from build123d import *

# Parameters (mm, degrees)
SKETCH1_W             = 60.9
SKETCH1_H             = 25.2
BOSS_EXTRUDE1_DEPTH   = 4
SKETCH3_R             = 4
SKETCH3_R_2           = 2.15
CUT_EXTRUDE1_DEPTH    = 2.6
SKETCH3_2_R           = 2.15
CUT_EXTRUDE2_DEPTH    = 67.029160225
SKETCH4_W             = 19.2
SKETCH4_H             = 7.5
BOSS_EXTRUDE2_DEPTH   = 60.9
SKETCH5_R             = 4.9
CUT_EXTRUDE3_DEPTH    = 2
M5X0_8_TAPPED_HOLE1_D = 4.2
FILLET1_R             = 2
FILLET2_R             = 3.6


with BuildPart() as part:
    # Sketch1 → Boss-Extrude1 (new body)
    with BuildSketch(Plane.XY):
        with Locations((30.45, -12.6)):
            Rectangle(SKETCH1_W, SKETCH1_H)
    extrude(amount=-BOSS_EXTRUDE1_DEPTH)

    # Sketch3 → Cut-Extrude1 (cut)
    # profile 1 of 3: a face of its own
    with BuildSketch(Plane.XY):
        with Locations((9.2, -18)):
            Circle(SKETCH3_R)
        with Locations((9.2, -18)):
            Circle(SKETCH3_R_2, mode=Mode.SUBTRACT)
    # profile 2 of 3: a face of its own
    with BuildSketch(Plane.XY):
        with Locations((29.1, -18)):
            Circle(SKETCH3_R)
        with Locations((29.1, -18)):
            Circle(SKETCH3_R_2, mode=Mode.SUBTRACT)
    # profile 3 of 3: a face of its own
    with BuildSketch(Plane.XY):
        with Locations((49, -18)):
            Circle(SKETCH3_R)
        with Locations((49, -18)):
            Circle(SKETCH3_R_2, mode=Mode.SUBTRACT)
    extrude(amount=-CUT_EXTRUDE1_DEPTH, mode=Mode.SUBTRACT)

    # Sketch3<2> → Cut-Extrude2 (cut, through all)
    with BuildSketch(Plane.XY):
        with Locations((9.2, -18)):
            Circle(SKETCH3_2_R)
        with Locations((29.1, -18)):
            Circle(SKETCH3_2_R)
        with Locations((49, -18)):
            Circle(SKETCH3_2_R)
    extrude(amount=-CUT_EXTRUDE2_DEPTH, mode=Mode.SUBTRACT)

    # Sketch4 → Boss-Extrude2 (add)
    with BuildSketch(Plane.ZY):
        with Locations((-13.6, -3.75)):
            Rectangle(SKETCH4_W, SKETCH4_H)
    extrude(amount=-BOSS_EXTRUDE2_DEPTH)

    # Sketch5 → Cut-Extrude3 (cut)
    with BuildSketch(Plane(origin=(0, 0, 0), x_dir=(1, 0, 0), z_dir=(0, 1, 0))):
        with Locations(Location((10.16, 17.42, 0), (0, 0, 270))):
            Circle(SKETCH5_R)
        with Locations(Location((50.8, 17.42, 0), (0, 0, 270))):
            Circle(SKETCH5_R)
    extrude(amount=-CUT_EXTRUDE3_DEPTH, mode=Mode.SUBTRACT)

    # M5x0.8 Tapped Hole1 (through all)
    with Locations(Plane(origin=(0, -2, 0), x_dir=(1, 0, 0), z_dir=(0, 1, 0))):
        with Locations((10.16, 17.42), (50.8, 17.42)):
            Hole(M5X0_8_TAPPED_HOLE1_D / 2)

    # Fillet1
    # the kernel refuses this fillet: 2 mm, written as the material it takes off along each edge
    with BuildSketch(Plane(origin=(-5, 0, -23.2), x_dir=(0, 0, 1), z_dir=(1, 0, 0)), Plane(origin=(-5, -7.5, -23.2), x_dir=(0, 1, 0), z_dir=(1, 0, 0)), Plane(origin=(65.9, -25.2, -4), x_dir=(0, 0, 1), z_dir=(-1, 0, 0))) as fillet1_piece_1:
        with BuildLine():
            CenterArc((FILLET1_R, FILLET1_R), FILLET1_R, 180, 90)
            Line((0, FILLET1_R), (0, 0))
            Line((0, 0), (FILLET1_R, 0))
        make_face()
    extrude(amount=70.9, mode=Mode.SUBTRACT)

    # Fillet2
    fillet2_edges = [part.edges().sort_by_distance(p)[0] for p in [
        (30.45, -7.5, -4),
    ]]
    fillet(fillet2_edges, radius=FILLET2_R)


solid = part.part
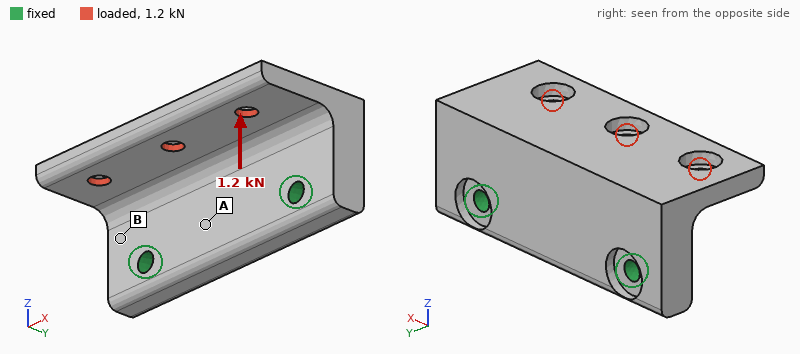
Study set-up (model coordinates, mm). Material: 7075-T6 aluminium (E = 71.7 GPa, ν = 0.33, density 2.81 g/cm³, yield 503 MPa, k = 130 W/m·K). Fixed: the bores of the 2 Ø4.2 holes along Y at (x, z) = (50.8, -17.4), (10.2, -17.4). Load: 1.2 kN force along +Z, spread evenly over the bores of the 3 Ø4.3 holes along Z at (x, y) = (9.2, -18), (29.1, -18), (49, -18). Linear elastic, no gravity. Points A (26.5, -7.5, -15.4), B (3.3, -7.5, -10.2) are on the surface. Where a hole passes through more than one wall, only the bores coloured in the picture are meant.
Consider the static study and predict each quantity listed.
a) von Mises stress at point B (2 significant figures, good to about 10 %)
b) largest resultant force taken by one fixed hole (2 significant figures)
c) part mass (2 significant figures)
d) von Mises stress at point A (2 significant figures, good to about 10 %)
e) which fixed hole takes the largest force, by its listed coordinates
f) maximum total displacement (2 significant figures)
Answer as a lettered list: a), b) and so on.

a) 35 MPa
b) 660 N
c) 39 g
d) 14 MPa
e) (10.2, -17.4)
f) 0.11 mm
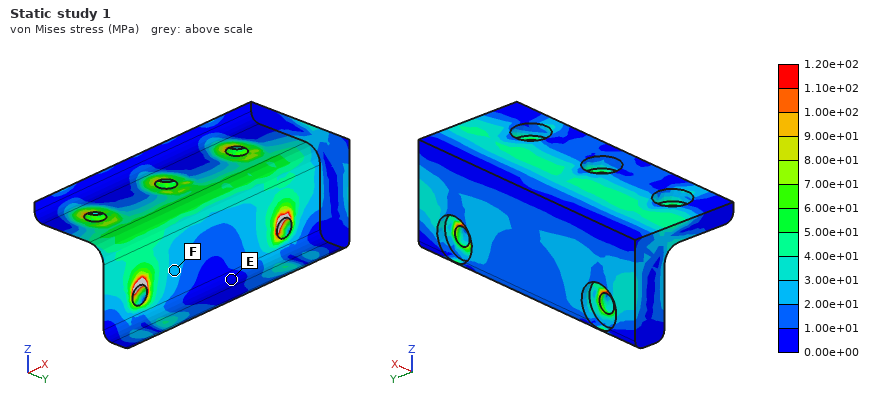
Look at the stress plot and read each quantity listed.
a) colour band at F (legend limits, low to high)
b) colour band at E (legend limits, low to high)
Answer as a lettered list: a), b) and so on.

a) 2.00e+01 to 3.00e+01 MPa
b) 0.00e+00 to 1.00e+01 MPa
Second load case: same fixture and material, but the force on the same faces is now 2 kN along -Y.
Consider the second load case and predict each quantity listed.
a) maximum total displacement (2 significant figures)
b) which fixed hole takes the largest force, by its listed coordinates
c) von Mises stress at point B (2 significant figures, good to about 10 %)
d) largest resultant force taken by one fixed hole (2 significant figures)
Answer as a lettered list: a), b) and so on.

a) 78 µm
b) (10.2, -17.4)
c) 33 MPa
d) 1.1 kN
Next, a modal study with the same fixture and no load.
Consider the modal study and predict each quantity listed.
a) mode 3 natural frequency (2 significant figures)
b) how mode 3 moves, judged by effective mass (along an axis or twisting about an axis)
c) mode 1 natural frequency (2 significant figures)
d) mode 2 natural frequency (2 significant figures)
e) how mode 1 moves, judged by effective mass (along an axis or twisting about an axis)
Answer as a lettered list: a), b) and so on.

a) 12 kHz
b) along Y
c) 5500 Hz
d) 8300 Hz
e) along Y
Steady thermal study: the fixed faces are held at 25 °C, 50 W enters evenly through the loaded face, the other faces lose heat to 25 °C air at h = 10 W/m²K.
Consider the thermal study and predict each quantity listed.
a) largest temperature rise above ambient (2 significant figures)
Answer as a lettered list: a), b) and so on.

a) 53 K
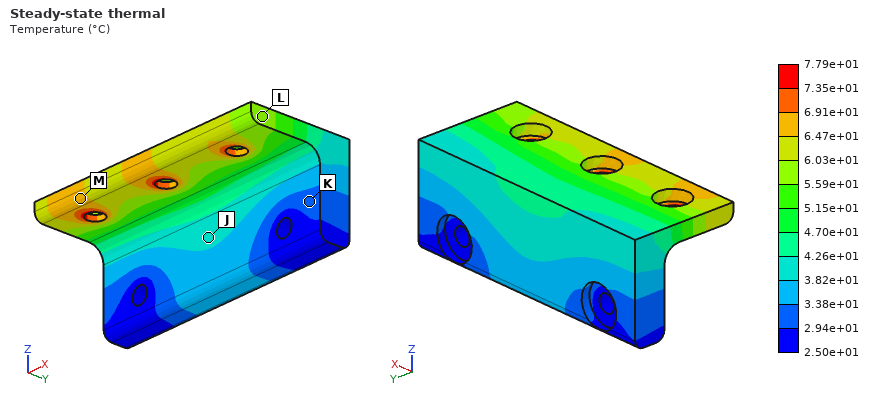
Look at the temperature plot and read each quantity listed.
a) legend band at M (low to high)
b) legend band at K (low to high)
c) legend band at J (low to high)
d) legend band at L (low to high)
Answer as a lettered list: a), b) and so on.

a) 6.47e+01 to 6.91e+01 °C
b) 2.94e+01 to 3.38e+01 °C
c) 3.82e+01 to 4.26e+01 °C
d) 5.59e+01 to 6.03e+01 °C
